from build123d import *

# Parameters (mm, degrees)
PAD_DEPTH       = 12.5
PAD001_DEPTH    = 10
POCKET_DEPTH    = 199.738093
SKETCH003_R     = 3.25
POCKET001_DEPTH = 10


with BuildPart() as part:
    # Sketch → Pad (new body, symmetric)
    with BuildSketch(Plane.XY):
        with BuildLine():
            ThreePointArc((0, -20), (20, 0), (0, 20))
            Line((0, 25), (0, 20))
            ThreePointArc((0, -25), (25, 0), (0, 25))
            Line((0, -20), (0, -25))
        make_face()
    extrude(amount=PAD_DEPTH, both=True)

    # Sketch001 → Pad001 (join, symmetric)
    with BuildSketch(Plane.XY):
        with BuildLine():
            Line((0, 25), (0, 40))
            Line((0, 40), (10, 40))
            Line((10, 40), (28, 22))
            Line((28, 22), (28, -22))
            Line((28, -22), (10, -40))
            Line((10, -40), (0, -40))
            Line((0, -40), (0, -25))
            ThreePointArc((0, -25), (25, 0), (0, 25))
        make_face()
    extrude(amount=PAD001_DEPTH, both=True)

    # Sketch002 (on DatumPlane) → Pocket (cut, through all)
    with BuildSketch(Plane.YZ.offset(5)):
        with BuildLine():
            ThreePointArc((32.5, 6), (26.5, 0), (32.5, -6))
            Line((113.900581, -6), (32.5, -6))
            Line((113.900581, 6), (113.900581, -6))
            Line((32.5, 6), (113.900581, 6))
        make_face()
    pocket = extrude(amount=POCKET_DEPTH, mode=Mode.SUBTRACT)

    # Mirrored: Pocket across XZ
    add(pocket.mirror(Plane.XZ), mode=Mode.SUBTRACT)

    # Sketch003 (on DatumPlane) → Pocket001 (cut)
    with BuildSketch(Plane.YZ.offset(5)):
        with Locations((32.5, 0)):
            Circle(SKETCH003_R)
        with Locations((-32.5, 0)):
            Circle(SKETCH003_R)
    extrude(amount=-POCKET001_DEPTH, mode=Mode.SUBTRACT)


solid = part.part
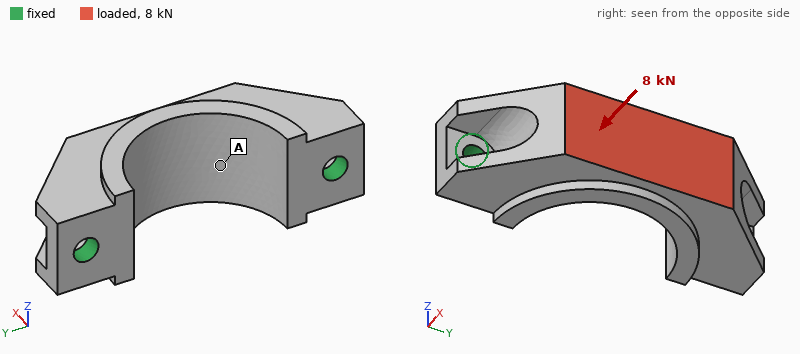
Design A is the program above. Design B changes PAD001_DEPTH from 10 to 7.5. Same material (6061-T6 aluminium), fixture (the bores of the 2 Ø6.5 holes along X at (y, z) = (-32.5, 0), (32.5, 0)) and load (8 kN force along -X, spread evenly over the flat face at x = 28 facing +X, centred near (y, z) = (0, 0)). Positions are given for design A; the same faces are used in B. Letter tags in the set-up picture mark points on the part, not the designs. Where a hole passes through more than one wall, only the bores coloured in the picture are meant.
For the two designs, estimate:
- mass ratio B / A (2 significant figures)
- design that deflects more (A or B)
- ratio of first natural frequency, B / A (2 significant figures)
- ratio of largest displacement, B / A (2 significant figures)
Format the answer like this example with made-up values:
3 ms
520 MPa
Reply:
0.80
B
1.00
1.1
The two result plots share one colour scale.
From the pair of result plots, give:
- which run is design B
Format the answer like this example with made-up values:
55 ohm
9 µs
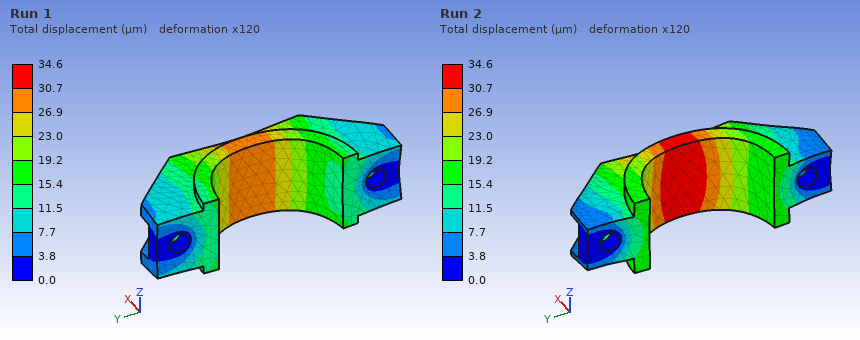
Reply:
Run 2
